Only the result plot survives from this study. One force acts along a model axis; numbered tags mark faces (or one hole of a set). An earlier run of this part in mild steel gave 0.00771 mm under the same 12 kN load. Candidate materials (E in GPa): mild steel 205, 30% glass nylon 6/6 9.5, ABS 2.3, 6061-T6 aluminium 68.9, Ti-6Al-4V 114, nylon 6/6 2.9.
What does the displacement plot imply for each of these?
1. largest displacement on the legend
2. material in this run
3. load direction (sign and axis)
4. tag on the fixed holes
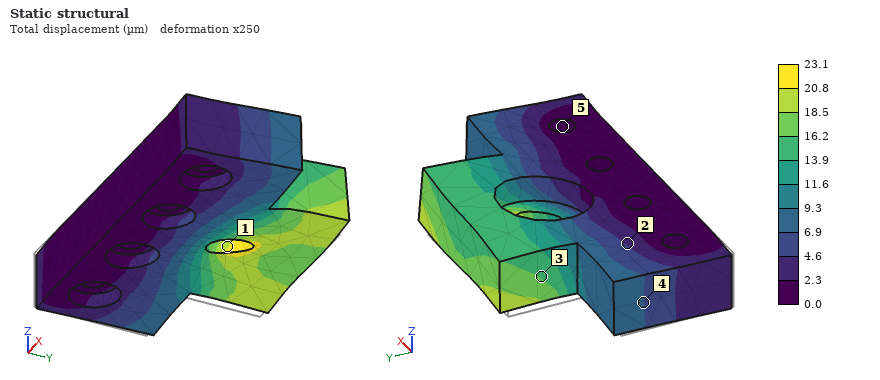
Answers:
23.1 µm
6061-T6 aluminium
+X
5
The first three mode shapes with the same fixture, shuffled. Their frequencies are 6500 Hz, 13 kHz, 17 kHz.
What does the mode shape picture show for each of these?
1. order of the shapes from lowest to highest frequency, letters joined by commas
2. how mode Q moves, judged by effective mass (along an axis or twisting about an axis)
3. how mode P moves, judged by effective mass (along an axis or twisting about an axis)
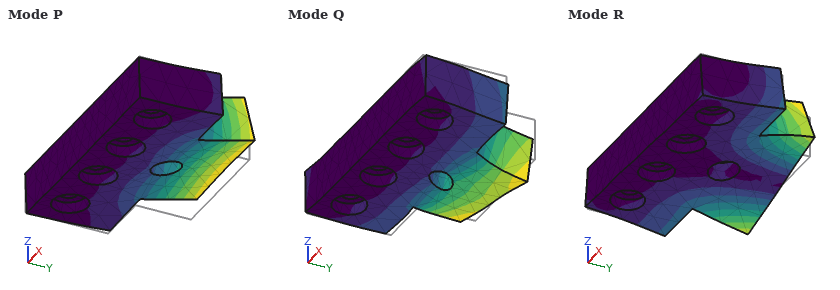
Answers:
P, R, Q
along X
along Z
